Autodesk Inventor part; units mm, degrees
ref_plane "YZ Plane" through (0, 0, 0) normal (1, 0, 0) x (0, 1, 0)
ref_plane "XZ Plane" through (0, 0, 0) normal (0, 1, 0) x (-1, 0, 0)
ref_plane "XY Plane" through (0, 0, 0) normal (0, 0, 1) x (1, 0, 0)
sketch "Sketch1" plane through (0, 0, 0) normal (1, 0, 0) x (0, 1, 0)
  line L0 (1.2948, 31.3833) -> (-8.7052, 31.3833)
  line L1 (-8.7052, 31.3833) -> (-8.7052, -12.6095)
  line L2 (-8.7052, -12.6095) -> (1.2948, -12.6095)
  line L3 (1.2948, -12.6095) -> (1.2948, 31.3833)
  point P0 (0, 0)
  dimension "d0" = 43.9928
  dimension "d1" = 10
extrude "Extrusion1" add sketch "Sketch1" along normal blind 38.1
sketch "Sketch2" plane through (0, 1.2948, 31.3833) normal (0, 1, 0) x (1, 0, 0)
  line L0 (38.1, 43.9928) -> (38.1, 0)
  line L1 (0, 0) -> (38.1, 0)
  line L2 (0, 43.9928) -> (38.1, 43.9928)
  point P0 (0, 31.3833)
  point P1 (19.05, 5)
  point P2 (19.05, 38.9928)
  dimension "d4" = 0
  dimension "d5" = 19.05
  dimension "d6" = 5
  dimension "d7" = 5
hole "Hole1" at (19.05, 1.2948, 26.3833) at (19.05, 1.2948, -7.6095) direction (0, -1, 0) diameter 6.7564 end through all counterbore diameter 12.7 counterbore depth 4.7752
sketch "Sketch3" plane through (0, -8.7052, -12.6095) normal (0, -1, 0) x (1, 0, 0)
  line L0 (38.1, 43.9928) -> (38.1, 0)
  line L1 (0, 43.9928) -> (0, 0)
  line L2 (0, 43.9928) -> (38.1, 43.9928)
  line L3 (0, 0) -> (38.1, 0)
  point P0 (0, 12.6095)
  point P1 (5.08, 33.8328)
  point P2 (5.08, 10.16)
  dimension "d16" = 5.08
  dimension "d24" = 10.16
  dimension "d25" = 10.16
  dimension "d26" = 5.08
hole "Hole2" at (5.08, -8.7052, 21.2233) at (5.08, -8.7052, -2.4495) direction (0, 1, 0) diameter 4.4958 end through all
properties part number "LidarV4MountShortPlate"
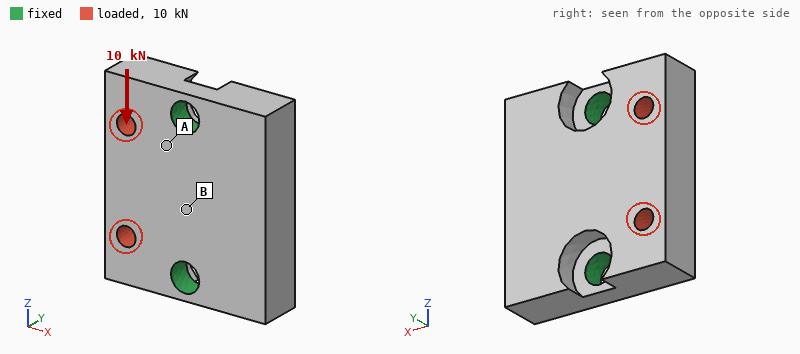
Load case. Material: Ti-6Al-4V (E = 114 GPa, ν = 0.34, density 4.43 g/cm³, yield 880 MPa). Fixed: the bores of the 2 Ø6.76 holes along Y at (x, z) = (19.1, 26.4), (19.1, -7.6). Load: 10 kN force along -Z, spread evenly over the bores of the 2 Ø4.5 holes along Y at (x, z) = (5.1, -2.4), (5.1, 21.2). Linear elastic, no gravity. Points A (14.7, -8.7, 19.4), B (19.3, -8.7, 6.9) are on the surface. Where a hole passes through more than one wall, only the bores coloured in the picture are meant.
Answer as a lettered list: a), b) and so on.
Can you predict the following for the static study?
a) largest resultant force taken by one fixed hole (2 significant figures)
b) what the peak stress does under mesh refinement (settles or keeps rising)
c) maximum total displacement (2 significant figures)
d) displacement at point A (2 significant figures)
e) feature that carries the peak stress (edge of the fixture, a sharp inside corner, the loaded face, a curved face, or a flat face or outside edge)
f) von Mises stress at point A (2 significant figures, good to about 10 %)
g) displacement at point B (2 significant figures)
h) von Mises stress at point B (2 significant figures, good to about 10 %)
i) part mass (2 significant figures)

a) 6.2 kN
b) keeps rising
c) 18 µm
d) 3.8 µm
e) edge of the fixture
f) 76 MPa
g) 3.1 µm
h) 25 MPa
i) 66 g
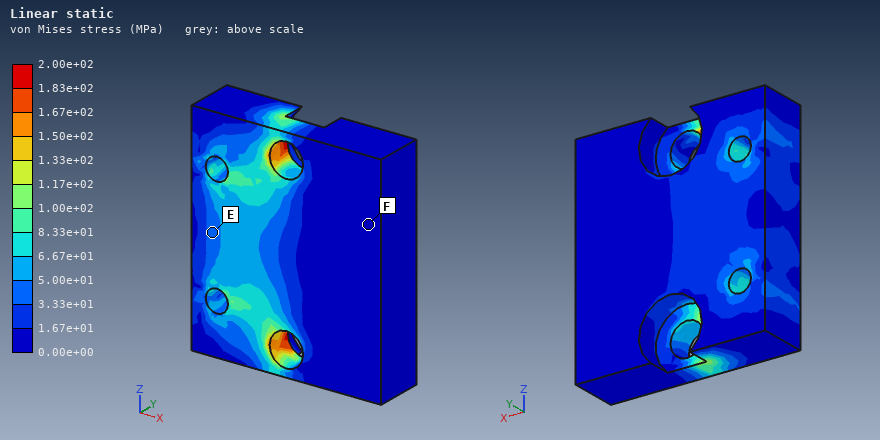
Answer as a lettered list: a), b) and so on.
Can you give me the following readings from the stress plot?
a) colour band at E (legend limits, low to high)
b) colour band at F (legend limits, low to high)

a) 3.33e+01 to 5.00e+01 MPa
b) 0.00e+00 to 1.67e+01 MPa
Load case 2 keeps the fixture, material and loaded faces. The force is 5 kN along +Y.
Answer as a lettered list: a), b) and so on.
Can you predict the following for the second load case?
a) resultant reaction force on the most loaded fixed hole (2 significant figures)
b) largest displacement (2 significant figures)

a) 2.8 kN
b) 72 µm
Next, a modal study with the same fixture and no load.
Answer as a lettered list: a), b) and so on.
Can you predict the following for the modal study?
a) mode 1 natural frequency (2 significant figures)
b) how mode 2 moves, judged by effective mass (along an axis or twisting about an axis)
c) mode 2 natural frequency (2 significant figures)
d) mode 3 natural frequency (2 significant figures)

a) 8700 Hz
b) along Y
c) 15 kHz
d) 20 kHz
